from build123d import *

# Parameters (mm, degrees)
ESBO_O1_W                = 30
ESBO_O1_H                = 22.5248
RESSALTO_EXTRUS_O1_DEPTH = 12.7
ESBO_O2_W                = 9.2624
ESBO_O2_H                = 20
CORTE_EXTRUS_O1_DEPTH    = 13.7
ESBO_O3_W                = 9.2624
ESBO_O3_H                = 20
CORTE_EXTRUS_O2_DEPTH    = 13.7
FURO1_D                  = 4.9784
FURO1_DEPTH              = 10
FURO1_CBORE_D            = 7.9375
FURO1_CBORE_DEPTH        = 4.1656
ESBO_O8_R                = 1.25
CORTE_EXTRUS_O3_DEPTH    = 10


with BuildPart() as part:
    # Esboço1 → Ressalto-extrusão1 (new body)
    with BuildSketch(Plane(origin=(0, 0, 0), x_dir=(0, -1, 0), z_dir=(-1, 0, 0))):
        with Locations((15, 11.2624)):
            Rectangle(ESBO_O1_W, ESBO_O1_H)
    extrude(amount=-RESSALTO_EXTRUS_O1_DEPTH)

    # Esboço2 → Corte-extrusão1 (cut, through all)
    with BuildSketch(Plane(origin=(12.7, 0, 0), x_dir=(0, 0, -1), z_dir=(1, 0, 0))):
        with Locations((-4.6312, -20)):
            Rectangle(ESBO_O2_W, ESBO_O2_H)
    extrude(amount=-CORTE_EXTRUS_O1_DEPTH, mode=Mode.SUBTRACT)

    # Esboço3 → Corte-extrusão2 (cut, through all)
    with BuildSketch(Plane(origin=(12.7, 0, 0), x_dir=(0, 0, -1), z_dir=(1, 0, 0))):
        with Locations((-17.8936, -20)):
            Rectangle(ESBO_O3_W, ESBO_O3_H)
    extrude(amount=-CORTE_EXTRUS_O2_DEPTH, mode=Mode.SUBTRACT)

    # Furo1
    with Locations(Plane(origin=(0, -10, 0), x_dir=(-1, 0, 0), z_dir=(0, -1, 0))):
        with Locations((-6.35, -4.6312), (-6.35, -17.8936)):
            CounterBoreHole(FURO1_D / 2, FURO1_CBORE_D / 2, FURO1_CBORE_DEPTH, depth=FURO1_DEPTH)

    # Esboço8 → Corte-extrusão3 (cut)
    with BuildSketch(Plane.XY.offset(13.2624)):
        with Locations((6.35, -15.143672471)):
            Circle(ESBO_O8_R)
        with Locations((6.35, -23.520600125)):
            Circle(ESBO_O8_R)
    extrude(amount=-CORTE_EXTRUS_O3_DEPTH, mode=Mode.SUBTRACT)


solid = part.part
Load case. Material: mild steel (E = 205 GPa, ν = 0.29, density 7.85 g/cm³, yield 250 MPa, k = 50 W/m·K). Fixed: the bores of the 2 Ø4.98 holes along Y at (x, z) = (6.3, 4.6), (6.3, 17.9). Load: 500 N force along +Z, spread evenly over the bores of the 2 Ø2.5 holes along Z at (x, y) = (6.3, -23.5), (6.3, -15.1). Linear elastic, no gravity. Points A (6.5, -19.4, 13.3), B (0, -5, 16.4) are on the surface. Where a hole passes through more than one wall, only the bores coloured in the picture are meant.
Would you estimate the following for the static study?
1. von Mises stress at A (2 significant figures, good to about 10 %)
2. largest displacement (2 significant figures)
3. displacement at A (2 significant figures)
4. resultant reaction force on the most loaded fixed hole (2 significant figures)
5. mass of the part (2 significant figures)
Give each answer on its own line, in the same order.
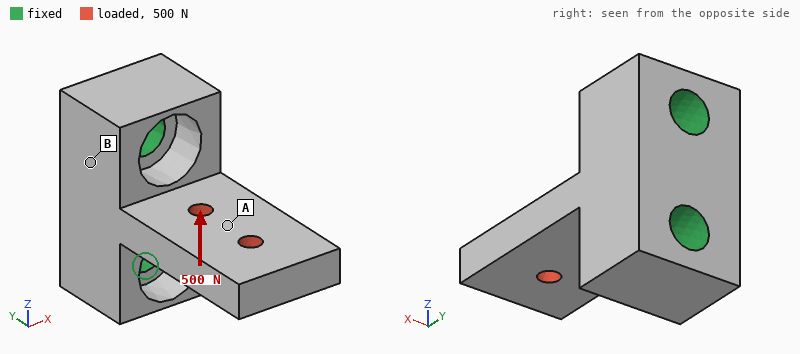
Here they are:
35 MPa
47 µm
19 µm
670 N
25 g
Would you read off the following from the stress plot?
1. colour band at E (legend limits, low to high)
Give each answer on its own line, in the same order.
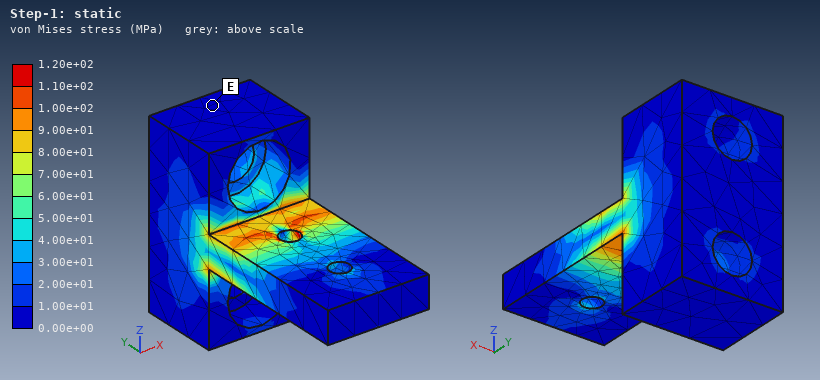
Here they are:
0.00e+00 to 1.00e+01 MPa
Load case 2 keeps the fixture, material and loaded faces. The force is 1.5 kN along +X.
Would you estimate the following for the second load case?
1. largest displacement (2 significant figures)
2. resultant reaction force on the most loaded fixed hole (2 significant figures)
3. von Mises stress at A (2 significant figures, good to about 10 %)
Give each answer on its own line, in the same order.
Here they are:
39 µm
750 N
56 MPa
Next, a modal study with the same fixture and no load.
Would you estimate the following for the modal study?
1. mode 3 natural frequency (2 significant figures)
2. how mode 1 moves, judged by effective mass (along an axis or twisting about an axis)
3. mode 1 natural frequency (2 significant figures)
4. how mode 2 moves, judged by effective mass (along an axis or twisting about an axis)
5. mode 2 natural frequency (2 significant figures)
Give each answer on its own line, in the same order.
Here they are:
21 kHz
along Z
6800 Hz
along X
13 kHz
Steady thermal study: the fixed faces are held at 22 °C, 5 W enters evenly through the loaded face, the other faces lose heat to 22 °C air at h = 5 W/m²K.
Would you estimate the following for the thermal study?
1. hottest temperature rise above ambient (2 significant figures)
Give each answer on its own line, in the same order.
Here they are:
29 K
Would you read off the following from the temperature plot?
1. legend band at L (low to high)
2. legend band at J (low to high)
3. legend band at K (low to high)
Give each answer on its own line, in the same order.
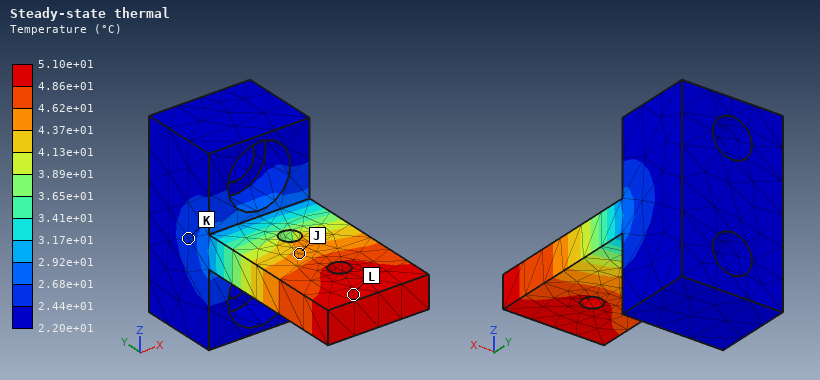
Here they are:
4.86e+01 to 5.10e+01 °C
4.37e+01 to 4.62e+01 °C
2.44e+01 to 2.68e+01 °C
